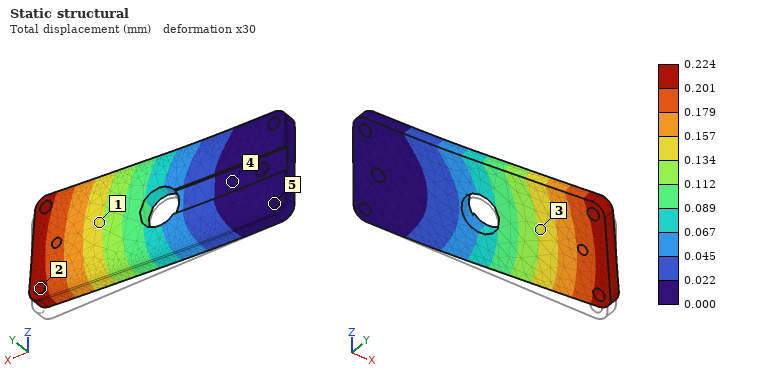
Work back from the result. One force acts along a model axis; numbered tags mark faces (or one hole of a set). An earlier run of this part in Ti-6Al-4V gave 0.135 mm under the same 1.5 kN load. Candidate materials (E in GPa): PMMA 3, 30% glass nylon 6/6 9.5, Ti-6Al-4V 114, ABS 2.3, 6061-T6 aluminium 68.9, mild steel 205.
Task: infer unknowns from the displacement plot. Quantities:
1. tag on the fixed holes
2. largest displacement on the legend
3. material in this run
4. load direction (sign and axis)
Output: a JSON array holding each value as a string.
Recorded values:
["5", "0.224 mm", "6061-T6 aluminium", "+Z"]
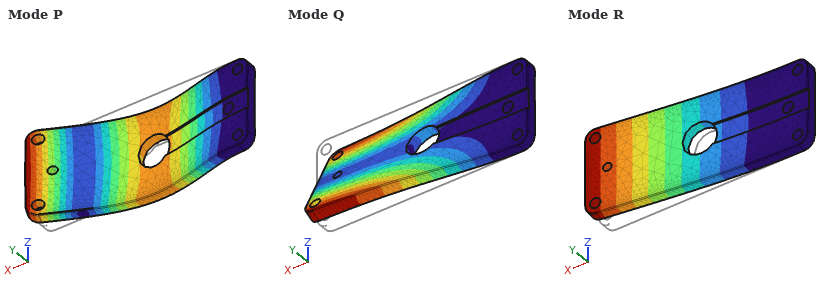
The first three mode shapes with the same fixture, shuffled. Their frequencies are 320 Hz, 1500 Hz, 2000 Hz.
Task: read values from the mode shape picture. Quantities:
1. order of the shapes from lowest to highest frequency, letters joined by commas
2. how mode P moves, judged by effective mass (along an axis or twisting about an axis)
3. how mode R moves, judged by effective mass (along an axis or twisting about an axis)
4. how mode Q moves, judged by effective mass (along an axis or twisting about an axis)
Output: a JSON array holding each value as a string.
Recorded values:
["R, Q, P", "along Y", "along Y", "twisting about X"]
